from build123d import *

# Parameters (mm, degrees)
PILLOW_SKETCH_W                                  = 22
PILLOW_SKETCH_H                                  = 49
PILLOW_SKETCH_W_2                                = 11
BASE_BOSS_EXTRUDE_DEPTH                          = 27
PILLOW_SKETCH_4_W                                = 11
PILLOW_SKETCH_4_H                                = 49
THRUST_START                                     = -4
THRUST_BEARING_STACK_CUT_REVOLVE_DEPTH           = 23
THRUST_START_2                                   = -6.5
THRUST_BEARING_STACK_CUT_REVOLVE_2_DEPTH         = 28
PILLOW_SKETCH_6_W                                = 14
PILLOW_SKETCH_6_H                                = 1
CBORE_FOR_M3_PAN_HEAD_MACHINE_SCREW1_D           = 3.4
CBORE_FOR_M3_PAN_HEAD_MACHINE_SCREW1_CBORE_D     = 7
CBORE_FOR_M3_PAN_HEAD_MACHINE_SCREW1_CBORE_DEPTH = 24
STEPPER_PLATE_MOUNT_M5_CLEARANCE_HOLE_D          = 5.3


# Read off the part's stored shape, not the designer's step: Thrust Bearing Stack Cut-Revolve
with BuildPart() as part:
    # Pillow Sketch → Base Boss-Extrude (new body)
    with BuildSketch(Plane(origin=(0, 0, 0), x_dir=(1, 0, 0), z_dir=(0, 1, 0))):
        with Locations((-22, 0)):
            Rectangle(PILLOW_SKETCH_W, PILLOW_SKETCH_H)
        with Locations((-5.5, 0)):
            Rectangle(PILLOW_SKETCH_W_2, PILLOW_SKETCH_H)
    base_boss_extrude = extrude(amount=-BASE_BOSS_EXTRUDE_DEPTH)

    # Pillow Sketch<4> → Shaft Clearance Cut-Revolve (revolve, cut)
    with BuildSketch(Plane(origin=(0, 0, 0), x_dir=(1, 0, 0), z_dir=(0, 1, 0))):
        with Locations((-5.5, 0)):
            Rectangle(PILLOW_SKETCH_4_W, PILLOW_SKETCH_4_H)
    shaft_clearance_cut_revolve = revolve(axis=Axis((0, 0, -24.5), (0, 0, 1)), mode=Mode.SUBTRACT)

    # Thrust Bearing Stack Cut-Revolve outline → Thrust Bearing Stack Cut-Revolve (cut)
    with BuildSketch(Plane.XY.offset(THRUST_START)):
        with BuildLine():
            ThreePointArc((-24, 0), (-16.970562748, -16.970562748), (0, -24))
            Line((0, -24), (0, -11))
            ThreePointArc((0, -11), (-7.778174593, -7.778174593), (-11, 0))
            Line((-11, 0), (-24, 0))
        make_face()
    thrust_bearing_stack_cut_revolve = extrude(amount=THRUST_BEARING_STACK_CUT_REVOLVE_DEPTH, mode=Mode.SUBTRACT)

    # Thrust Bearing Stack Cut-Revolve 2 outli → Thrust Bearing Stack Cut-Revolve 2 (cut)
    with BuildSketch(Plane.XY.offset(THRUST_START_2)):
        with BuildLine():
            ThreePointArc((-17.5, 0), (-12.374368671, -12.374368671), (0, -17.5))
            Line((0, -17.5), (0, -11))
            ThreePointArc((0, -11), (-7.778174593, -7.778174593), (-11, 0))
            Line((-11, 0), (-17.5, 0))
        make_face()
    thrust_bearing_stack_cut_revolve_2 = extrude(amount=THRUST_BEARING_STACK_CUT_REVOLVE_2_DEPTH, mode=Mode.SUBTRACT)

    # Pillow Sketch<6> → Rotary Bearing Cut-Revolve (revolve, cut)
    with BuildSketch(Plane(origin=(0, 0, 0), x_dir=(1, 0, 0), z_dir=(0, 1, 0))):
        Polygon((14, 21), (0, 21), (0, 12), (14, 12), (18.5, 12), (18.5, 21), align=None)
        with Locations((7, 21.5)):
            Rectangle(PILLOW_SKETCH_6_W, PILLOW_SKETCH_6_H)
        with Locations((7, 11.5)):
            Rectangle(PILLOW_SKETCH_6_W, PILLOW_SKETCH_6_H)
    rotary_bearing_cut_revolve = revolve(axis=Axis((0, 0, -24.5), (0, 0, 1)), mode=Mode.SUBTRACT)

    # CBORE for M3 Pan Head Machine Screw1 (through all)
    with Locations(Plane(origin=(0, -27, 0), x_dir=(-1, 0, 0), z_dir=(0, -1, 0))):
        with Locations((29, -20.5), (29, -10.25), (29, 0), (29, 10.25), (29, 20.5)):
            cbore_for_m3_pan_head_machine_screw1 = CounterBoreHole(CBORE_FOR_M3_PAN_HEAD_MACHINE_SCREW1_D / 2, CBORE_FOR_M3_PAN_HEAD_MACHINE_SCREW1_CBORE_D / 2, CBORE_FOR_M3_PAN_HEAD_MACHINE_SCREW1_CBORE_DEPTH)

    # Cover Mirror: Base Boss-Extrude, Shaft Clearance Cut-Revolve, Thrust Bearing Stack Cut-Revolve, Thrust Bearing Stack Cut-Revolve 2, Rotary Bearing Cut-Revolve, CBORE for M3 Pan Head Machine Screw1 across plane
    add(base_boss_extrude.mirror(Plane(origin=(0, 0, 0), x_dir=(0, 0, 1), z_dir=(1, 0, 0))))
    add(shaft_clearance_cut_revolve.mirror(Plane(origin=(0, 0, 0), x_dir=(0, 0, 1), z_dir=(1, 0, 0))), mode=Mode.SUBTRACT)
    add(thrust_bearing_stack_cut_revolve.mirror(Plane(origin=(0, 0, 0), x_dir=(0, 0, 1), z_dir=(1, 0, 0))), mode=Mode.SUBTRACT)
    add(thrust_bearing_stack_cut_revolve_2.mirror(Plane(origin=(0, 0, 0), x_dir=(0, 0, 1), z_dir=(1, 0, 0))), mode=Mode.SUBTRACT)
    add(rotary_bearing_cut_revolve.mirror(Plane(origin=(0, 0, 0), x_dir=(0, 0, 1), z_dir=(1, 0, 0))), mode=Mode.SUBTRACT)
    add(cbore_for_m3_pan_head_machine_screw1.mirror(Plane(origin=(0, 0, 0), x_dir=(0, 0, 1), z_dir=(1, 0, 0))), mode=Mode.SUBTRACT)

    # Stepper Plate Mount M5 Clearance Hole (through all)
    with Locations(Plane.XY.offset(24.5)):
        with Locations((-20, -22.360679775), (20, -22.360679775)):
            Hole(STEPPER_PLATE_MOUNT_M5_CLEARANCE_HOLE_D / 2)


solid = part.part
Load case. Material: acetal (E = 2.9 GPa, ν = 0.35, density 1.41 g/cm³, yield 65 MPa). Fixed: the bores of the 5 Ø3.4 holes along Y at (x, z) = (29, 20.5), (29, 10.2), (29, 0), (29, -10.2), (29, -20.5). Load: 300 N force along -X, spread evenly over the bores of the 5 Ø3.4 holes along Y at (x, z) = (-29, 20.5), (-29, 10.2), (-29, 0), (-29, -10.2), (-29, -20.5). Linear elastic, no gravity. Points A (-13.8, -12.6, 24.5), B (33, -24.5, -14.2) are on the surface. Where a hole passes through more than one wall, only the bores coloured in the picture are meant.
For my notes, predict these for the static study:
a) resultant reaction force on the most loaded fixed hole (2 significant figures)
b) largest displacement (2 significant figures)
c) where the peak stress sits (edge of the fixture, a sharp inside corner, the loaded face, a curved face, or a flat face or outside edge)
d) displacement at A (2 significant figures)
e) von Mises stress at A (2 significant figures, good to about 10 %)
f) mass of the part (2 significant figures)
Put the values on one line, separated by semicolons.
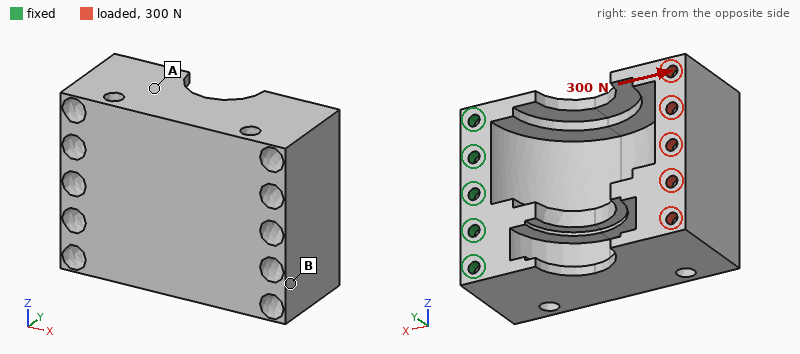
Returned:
99 N; 0.38 mm; a curved face; 0.14 mm; 3.3 MPa; 64 g
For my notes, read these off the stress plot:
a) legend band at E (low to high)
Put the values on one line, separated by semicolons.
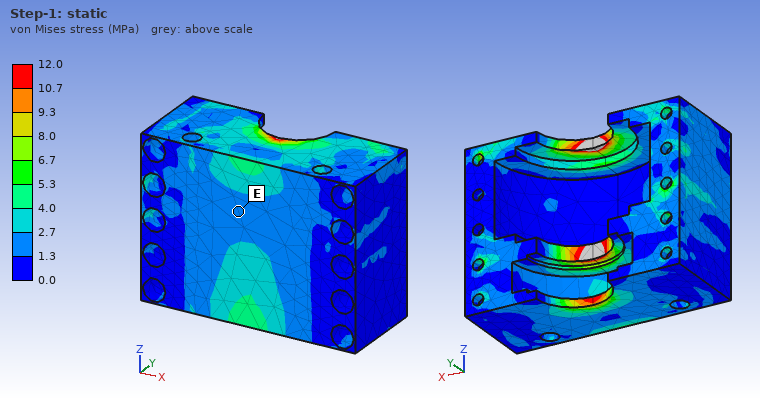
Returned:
1.3 to 2.7 MPa
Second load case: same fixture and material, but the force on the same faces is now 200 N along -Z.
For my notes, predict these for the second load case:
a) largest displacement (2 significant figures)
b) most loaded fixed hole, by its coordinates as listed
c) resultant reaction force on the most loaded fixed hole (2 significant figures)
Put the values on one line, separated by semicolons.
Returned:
0.88 mm; (29, -20.5); 350 N
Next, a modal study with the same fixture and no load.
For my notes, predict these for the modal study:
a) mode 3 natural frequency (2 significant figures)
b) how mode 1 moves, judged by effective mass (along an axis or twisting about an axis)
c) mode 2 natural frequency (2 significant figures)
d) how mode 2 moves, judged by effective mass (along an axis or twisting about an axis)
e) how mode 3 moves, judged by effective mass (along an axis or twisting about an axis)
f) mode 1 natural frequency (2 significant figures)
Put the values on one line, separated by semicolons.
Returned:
1500 Hz; along Y; 630 Hz; along Z; along X; 290 Hz
